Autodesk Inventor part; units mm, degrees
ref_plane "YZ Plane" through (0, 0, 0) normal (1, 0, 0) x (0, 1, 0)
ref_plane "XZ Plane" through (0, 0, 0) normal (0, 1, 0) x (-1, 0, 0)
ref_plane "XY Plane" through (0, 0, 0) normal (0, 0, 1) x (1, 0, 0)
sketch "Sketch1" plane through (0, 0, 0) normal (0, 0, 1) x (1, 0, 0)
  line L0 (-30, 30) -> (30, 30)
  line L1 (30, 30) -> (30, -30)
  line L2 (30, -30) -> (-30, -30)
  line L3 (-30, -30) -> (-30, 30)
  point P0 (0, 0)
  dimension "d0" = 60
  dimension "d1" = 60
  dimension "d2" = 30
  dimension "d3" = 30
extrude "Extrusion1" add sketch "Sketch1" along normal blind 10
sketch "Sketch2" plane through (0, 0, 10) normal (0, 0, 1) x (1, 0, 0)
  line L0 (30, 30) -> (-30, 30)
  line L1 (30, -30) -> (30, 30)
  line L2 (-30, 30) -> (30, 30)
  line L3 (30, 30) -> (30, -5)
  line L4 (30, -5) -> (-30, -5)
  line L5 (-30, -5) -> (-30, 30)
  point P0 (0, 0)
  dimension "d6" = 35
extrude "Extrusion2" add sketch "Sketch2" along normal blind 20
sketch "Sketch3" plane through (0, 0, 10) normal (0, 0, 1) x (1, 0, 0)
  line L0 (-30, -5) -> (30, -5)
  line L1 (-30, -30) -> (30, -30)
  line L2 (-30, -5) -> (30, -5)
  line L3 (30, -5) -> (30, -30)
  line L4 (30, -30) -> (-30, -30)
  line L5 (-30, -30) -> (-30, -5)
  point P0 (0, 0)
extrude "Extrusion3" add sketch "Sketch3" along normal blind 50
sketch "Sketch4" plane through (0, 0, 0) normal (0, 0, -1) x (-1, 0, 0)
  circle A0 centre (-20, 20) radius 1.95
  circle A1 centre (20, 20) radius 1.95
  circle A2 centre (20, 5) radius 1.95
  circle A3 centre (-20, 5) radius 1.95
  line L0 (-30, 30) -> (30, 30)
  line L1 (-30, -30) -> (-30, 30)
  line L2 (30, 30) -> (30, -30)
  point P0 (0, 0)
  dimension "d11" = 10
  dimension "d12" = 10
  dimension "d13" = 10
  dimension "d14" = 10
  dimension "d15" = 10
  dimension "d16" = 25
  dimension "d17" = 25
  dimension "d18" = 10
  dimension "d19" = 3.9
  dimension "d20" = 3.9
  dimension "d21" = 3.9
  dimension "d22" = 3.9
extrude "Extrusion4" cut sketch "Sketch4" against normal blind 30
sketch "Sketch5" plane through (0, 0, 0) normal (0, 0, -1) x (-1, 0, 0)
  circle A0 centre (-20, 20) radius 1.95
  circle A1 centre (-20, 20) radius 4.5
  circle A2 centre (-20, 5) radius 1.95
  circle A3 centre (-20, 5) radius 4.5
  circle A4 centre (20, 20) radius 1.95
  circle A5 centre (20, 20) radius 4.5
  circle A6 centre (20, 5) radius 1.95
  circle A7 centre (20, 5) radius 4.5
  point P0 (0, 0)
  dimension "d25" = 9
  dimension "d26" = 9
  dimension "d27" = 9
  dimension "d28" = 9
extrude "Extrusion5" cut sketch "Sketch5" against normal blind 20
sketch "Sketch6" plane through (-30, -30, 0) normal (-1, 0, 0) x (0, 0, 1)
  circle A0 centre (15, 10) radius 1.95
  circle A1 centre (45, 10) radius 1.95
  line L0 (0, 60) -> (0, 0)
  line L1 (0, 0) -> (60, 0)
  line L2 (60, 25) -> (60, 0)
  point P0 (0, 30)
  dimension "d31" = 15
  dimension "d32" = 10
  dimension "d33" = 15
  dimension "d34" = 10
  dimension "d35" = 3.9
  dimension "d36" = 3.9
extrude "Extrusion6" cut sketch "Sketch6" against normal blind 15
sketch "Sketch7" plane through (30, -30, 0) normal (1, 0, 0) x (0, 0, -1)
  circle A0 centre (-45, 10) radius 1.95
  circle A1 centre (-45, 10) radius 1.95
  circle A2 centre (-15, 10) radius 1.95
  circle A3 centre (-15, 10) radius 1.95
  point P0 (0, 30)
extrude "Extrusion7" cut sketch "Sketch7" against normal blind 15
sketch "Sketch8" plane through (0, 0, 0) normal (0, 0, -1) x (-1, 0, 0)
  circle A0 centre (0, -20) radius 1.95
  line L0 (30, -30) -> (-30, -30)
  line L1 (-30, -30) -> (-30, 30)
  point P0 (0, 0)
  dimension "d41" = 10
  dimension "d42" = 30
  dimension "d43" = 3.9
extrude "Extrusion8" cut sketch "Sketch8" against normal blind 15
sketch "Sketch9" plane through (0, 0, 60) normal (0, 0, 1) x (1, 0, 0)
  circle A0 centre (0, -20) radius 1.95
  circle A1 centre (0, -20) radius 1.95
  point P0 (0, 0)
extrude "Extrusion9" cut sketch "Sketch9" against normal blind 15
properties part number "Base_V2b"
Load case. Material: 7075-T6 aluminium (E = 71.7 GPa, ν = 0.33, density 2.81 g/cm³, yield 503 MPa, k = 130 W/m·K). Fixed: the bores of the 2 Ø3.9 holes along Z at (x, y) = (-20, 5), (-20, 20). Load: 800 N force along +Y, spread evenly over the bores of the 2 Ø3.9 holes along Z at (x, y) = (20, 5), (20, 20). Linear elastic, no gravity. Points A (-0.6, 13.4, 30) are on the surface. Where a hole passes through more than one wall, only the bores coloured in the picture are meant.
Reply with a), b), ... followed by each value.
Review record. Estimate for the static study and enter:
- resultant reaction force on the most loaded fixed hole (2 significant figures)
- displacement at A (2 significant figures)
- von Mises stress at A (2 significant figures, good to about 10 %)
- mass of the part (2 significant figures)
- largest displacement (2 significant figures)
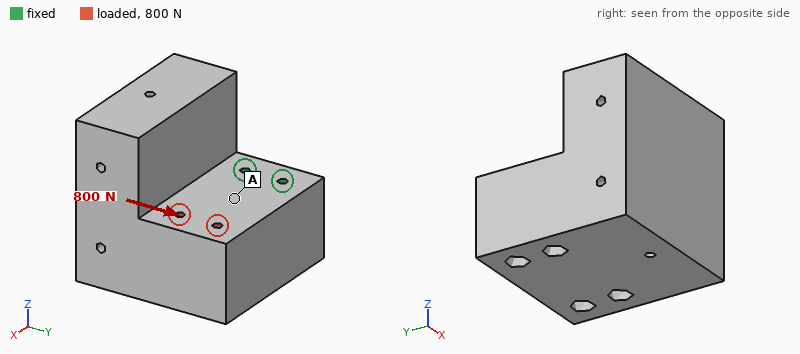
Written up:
a) 1.8 kN
b) 5.1 µm
c) 5.0 MPa
d) 410 g
e) 17 µm
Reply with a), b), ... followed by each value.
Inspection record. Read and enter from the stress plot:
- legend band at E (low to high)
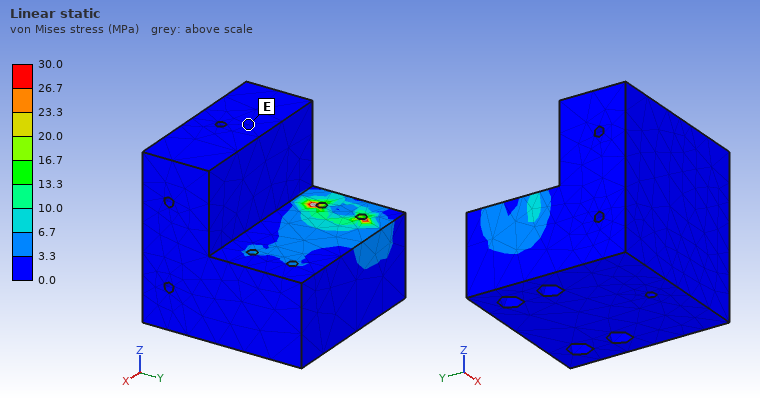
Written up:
a) 0.0 to 3.3 MPa
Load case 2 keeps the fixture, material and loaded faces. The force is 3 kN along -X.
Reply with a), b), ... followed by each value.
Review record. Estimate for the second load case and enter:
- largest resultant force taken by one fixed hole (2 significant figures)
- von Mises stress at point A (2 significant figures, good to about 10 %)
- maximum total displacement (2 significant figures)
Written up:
a) 1.5 kN
b) 8.3 MPa
c) 6.8 µm
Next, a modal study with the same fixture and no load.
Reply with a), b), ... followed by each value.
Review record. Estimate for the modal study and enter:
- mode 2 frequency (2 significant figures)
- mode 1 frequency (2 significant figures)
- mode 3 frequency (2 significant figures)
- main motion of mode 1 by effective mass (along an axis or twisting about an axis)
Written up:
a) 2400 Hz
b) 1600 Hz
c) 3100 Hz
d) along Z
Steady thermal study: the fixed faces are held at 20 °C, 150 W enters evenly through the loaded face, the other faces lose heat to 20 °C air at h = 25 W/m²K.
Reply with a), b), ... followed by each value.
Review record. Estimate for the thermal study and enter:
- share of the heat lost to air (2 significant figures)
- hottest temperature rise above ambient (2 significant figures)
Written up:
a) 11 %
b) 66 K
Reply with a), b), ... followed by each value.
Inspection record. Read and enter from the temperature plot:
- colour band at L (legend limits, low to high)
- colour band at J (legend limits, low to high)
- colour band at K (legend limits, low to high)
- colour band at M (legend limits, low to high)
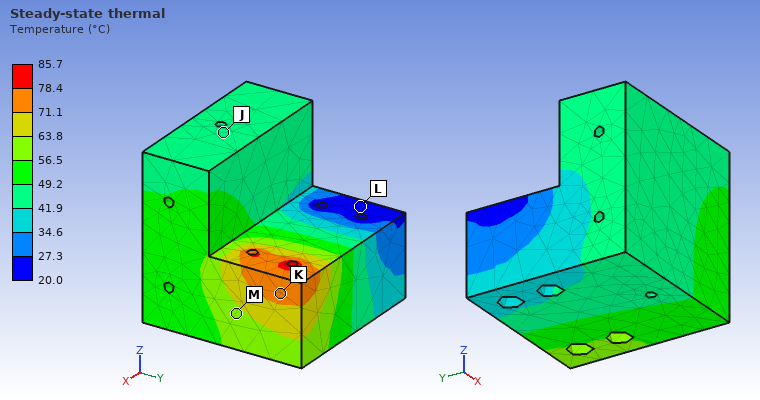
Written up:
a) 20.0 to 27.3 °C
b) 41.9 to 49.2 °C
c) 71.1 to 78.4 °C
d) 56.5 to 63.8 °C
